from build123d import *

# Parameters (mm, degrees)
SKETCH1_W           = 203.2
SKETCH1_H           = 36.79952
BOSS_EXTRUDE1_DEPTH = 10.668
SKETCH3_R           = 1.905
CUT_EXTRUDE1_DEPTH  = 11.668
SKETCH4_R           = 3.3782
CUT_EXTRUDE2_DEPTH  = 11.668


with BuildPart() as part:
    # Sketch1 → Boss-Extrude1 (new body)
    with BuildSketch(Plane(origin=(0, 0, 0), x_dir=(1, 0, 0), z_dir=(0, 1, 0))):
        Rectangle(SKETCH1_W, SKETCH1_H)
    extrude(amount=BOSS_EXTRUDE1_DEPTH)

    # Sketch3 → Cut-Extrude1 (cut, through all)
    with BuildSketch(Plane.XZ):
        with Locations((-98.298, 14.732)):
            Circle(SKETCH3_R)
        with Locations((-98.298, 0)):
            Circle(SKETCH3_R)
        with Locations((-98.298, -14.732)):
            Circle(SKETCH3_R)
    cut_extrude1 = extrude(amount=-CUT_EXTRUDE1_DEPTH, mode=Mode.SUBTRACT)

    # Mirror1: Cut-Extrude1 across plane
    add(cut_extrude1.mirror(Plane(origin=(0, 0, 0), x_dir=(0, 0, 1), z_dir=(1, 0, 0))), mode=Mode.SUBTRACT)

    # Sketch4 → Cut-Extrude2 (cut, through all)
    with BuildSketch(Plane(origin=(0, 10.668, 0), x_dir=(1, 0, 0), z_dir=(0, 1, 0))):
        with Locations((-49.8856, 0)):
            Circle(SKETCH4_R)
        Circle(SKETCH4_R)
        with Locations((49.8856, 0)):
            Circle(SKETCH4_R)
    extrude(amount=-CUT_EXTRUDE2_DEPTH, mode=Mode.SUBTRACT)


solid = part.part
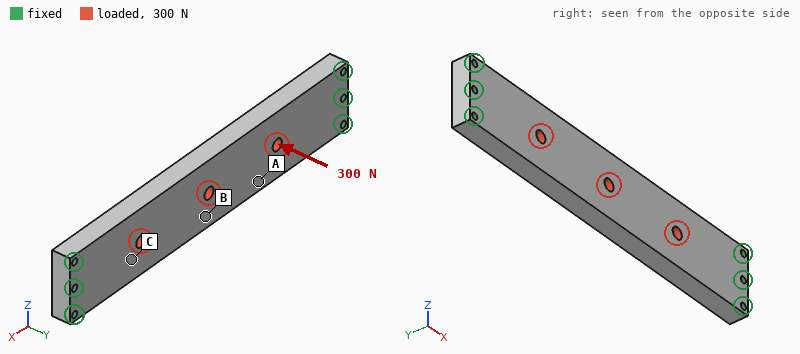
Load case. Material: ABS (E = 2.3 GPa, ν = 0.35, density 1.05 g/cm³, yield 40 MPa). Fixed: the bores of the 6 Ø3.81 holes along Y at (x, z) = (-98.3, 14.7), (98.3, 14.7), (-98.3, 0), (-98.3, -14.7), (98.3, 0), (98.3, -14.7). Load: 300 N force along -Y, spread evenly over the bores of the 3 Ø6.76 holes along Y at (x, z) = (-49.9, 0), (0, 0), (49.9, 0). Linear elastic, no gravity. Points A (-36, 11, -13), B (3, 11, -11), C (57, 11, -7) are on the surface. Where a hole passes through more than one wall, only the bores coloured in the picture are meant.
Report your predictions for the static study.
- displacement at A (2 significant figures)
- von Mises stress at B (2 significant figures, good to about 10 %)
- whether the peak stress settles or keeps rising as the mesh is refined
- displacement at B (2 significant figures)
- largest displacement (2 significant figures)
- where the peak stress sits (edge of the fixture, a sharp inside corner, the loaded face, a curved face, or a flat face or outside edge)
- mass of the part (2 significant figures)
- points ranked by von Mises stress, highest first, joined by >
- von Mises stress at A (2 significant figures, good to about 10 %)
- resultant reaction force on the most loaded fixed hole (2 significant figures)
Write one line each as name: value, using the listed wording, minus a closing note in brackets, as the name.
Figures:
displacement at A: 0.72 mm
von Mises stress at B: 5.4 MPa
whether the peak stress settles or keeps rising as the mesh is refined: keeps rising
displacement at B: 0.96 mm
largest displacement: 0.97 mm
where the peak stress sits: edge of the fixture
mass of the part: 82 g
points ranked by von Mises stress, highest first, joined by >: B > A > C
von Mises stress at A: 2.7 MPa
resultant reaction force on the most loaded fixed hole: 89 N
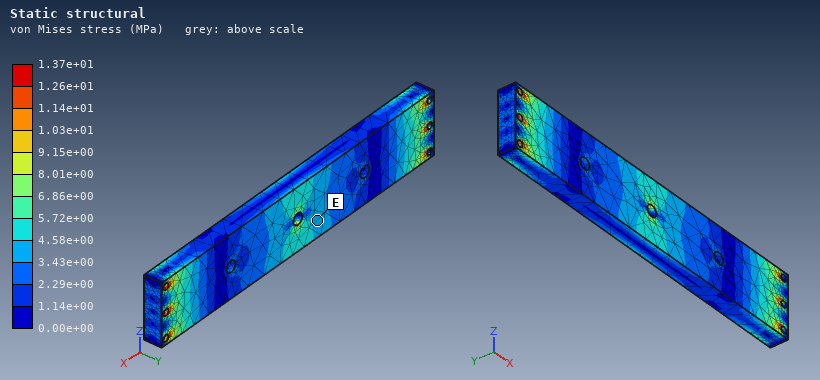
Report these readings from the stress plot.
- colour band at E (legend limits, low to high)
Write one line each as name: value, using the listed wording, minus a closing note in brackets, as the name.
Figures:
colour band at E: 3.43e+00 to 4.58e+00 MPa
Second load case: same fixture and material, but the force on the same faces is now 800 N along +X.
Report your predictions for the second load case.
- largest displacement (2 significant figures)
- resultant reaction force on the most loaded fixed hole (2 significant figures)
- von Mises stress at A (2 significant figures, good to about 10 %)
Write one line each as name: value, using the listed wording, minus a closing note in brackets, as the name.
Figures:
largest displacement: 33 µm
resultant reaction force on the most loaded fixed hole: 140 N
von Mises stress at A: 0.53 MPa
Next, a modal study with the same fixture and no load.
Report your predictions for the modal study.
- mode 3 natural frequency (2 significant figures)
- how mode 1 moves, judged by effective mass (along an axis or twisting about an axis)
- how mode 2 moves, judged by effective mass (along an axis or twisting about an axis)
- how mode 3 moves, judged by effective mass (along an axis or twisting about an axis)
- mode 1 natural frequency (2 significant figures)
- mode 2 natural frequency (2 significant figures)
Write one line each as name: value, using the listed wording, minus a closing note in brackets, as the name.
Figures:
mode 3 natural frequency: 1200 Hz
how mode 1 moves, judged by effective mass: along Y
how mode 2 moves, judged by effective mass: twisting about Z
how mode 3 moves, judged by effective mass: along Z
mode 1 natural frequency: 410 Hz
mode 2 natural frequency: 1100 Hz
